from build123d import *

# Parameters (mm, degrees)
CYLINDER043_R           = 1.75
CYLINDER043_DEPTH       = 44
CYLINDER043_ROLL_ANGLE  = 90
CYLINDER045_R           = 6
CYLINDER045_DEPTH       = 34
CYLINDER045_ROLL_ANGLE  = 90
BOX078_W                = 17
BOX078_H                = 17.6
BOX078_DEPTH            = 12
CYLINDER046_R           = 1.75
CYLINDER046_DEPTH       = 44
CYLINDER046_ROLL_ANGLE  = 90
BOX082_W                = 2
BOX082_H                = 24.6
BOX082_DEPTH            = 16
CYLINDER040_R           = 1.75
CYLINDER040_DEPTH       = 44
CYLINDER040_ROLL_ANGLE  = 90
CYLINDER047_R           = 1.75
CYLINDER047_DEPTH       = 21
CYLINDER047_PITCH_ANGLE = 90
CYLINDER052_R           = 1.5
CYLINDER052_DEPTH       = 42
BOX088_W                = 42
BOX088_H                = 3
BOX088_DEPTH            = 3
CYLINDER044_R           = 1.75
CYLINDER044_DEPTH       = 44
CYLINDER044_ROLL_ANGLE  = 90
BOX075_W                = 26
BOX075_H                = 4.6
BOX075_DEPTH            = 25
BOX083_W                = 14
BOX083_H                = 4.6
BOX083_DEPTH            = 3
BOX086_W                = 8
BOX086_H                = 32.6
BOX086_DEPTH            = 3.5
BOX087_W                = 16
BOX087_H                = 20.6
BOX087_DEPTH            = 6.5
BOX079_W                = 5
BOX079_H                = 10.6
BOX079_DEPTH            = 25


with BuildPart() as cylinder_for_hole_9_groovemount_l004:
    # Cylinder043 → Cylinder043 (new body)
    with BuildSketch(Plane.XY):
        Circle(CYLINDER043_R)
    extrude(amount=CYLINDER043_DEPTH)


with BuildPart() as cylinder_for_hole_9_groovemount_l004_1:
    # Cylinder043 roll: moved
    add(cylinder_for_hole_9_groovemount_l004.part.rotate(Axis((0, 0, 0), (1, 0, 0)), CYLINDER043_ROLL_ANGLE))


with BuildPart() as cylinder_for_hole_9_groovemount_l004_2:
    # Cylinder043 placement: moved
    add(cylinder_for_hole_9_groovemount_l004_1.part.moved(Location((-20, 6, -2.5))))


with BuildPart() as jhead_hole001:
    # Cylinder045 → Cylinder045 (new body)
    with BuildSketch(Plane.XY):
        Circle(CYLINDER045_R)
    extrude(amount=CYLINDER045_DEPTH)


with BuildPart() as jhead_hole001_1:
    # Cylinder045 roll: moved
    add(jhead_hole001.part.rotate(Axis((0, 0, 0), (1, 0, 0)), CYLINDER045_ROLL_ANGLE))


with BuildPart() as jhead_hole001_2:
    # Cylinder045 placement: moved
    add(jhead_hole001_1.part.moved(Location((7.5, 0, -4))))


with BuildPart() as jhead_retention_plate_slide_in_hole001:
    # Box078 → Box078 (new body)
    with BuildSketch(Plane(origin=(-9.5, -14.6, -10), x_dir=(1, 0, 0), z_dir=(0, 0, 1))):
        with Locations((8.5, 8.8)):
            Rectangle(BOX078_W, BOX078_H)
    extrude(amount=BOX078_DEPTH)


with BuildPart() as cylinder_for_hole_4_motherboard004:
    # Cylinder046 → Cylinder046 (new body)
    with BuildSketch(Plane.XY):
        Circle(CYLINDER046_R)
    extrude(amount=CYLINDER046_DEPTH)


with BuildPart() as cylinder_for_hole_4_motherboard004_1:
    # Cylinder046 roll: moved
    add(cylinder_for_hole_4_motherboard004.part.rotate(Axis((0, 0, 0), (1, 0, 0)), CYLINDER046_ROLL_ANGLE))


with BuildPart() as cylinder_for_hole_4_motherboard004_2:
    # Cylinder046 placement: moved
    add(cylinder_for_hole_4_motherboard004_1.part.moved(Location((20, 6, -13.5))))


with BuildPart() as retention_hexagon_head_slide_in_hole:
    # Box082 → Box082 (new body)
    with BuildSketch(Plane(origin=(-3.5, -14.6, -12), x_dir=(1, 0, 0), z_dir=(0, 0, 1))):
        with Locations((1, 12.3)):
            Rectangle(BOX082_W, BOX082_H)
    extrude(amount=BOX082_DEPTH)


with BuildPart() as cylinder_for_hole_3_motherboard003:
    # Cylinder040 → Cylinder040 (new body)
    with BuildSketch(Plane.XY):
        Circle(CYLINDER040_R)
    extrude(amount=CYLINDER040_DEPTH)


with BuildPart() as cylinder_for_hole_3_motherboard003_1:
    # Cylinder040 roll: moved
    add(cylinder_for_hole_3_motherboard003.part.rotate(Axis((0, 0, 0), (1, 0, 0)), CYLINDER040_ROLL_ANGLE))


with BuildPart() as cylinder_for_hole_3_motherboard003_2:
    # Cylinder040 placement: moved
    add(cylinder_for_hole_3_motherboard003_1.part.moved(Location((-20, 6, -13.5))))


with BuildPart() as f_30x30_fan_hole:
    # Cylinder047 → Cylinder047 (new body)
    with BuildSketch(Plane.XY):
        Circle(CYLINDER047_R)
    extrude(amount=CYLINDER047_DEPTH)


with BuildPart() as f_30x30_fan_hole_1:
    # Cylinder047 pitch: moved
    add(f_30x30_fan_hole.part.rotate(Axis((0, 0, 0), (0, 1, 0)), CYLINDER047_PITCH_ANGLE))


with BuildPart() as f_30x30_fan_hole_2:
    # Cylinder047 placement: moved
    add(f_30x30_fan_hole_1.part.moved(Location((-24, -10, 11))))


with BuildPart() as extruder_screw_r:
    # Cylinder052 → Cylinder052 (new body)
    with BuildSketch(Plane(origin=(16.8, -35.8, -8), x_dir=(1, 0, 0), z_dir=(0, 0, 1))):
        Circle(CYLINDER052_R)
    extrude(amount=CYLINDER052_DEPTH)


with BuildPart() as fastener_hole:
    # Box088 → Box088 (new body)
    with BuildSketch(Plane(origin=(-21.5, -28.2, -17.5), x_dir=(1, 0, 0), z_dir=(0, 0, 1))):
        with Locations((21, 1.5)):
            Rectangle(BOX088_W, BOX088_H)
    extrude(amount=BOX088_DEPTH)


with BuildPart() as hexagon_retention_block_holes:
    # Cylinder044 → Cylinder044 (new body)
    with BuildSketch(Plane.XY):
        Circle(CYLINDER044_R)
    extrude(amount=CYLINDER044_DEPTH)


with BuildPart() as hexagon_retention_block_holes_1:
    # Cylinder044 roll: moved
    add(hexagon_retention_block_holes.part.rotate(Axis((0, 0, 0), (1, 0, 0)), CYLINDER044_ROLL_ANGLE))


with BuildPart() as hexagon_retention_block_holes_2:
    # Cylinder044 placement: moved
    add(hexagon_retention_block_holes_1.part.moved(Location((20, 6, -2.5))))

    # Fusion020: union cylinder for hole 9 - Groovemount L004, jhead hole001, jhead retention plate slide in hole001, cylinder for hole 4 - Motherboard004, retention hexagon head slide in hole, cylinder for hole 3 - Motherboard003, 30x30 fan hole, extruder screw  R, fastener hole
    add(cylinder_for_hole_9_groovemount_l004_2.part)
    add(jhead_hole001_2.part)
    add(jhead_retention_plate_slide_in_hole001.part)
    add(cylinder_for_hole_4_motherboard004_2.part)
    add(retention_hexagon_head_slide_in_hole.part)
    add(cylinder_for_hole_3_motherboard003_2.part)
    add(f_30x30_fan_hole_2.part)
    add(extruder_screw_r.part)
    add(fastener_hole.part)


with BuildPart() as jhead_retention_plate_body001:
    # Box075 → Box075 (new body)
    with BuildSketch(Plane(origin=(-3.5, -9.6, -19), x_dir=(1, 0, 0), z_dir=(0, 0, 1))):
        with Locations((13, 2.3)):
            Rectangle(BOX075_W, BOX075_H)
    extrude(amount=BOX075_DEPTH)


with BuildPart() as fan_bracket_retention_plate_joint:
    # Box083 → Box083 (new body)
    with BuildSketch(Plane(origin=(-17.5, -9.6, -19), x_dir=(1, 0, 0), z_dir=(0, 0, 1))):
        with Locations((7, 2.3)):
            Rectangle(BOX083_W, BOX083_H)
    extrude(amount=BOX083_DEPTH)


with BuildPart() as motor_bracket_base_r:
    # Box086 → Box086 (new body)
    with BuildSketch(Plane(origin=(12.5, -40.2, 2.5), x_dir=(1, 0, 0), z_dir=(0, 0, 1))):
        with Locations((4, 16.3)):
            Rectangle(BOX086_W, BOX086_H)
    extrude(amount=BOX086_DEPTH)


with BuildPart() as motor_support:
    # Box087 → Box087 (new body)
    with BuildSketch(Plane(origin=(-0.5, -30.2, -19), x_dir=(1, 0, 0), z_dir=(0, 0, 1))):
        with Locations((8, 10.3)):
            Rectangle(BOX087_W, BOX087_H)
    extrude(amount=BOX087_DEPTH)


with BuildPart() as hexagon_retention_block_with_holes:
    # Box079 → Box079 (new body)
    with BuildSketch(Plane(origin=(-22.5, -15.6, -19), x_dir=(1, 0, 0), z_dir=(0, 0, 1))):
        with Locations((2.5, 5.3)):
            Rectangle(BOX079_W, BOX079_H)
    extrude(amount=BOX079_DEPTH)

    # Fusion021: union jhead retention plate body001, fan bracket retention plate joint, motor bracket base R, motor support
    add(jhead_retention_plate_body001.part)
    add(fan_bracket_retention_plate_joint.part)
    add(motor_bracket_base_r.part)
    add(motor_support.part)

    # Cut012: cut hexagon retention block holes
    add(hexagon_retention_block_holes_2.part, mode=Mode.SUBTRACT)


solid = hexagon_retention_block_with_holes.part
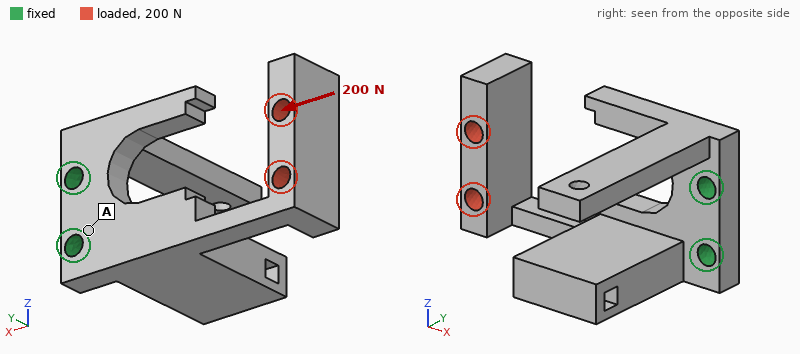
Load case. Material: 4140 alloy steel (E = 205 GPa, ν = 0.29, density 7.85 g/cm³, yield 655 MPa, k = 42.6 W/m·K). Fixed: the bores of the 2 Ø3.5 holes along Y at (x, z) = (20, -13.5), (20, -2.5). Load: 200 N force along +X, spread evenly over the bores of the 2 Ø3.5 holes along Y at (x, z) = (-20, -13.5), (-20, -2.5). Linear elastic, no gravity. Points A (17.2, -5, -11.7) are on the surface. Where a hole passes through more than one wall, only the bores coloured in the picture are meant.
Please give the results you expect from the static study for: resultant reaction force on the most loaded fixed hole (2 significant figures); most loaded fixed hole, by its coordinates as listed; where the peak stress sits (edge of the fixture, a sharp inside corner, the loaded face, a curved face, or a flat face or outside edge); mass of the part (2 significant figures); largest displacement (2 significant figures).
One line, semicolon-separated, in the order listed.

130 N; (20, -13.5); a flat face or outside edge; 48 g; 0.44 mm
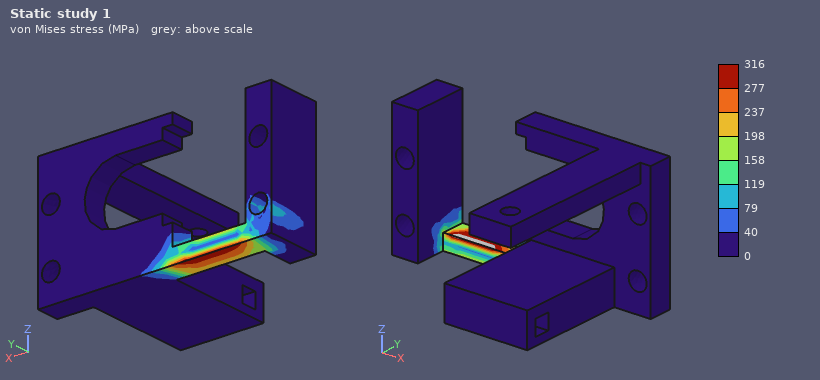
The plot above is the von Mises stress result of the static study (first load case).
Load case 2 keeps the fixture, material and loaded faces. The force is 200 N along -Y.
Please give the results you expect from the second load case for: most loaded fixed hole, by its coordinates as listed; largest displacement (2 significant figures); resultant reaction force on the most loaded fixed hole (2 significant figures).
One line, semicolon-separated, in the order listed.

(20, -13.5); 0.61 mm; 120 N
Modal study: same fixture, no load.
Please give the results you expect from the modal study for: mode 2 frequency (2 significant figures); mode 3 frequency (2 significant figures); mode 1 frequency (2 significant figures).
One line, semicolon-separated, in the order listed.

1100 Hz; 2600 Hz; 1100 Hz
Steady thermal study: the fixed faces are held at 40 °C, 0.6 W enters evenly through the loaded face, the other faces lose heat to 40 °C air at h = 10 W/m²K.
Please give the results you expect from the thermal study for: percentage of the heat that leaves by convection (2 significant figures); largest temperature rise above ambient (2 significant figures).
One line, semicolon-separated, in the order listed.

34 %; 19 K
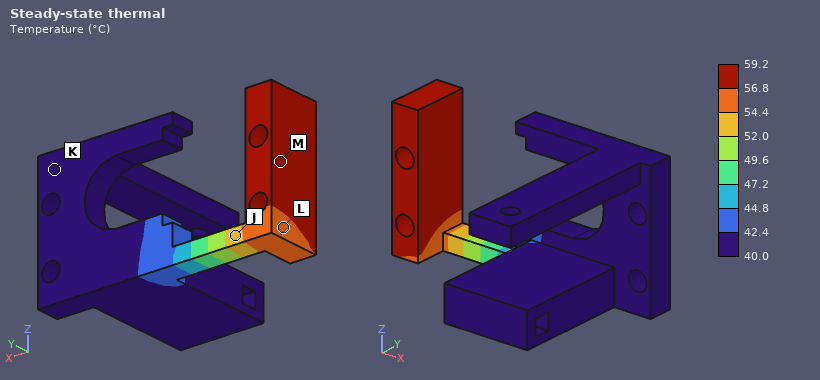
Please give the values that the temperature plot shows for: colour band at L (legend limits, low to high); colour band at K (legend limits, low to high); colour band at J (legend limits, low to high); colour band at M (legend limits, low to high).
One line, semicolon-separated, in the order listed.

54.4 to 56.8 °C; 40.0 to 42.4 °C; 52.0 to 54.4 °C; 56.8 to 59.2 °C
